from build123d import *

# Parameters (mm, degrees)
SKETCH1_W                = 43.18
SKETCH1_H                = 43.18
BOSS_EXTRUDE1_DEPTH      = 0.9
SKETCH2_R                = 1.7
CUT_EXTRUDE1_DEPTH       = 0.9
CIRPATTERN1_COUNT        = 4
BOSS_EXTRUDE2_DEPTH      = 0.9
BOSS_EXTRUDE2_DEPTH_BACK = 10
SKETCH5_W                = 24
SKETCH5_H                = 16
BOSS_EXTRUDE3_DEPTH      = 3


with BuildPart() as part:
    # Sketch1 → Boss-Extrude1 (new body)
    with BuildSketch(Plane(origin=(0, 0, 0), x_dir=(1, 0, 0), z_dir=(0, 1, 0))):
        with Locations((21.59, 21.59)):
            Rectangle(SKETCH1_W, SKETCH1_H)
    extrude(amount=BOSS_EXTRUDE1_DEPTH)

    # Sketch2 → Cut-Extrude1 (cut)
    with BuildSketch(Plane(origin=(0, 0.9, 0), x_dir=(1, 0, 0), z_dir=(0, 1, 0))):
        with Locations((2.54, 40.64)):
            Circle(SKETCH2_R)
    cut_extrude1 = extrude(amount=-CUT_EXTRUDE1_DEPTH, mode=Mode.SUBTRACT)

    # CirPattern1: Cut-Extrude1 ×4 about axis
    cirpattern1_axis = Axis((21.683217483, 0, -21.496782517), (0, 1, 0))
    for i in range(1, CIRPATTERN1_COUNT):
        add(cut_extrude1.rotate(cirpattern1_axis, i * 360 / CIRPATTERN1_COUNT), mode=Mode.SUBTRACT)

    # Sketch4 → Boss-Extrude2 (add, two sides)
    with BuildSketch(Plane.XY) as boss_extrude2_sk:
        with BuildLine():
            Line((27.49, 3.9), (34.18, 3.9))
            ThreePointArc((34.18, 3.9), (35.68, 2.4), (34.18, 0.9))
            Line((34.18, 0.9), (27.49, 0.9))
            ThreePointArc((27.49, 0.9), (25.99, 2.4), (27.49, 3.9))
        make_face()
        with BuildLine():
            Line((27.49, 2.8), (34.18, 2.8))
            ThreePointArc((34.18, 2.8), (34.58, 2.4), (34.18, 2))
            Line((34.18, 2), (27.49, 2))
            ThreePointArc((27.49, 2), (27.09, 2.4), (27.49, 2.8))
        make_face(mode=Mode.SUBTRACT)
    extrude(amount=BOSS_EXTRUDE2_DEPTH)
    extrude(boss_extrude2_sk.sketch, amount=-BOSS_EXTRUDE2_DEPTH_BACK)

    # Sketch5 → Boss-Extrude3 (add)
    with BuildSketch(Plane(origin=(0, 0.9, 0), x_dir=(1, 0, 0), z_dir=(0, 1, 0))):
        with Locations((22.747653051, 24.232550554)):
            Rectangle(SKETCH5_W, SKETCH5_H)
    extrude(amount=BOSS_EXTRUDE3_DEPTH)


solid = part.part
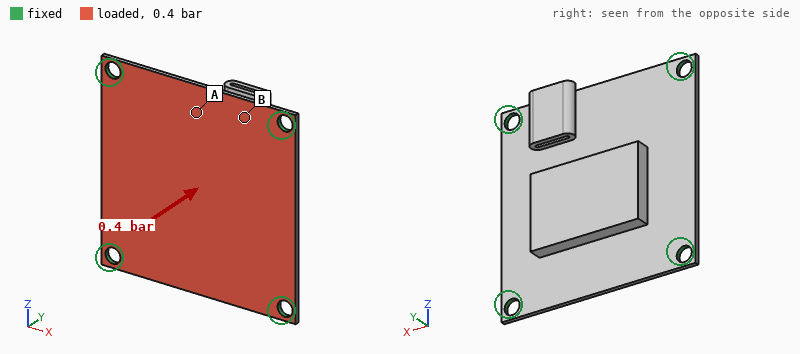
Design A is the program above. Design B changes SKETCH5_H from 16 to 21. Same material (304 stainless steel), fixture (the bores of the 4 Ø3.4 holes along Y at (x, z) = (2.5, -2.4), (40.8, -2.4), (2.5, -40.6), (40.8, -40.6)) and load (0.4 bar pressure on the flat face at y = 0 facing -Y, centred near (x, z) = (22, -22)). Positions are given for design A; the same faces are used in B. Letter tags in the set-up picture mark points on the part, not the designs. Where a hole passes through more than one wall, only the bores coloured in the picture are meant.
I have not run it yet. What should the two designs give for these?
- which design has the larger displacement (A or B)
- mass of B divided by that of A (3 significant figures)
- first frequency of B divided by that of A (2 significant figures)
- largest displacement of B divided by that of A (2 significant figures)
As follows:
A
1.12
1.1
0.78
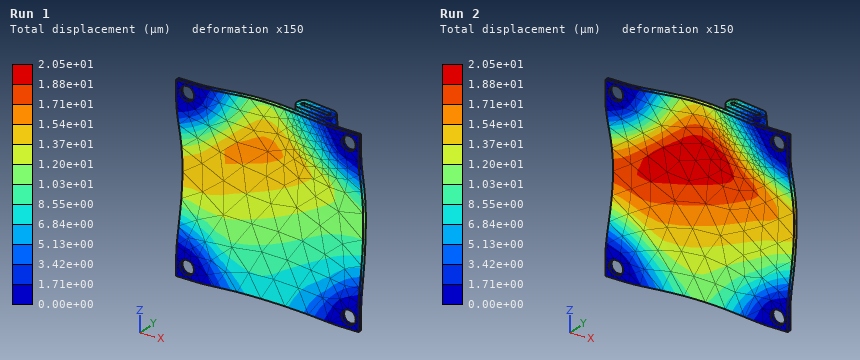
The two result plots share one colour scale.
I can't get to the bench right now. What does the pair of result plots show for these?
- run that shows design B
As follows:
Run 1
